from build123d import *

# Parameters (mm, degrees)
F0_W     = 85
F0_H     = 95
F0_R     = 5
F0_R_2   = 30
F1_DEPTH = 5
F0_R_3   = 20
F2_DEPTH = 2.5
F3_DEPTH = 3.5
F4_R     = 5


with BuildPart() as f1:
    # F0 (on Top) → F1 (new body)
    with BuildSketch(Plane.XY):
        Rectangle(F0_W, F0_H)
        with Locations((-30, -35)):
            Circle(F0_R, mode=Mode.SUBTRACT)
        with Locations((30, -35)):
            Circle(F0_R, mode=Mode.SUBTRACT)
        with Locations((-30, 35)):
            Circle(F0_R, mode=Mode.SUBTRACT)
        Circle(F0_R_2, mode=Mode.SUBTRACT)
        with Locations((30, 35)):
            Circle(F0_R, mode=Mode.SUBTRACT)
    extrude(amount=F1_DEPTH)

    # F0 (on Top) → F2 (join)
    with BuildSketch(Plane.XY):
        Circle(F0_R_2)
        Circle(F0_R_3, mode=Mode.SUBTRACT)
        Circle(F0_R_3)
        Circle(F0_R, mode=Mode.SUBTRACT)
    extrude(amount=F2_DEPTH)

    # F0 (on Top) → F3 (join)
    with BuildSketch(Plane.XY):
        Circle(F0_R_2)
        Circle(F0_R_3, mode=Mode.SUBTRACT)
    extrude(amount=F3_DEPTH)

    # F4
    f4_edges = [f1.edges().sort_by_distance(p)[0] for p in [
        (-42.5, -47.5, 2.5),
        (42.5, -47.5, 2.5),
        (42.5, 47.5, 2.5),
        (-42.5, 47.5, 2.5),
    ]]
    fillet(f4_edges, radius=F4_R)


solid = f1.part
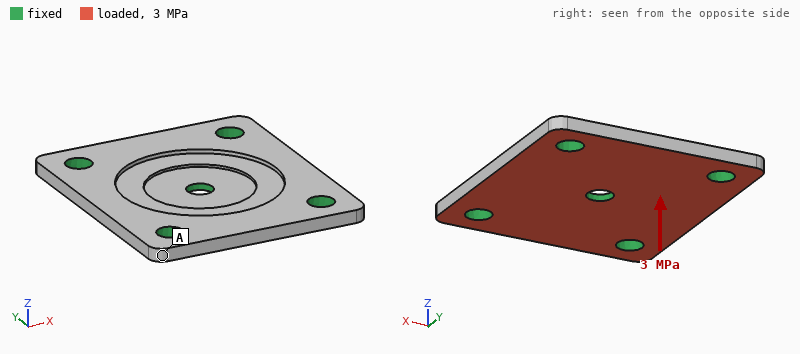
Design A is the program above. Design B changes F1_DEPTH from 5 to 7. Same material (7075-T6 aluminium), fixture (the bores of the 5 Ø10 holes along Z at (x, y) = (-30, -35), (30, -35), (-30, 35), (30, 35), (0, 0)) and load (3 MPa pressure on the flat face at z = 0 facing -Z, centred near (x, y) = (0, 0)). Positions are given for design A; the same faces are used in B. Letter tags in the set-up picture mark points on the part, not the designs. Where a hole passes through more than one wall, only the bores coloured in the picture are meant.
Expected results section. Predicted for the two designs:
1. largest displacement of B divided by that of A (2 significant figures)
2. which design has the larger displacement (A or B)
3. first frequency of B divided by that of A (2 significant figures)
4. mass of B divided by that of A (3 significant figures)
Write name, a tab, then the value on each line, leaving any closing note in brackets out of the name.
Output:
largest displacement of B divided by that of A	0.46
which design has the larger displacement	A
first frequency of B divided by that of A	1.3
mass of B divided by that of A	1.30
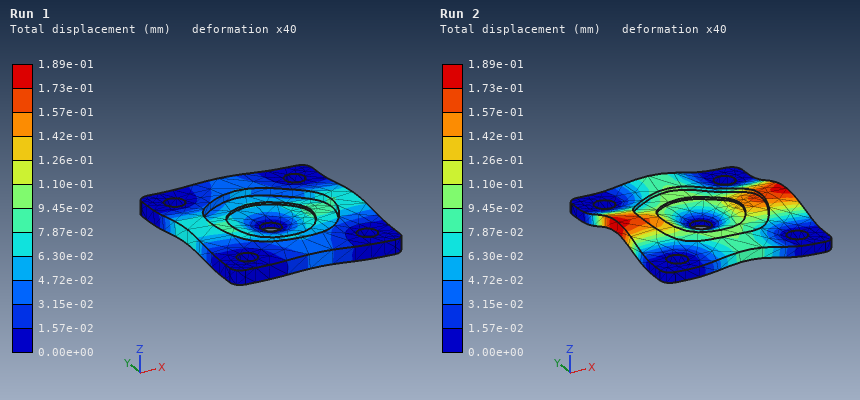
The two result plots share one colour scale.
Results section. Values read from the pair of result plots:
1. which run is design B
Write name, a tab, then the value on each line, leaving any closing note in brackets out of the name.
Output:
which run is design B	Run 1
